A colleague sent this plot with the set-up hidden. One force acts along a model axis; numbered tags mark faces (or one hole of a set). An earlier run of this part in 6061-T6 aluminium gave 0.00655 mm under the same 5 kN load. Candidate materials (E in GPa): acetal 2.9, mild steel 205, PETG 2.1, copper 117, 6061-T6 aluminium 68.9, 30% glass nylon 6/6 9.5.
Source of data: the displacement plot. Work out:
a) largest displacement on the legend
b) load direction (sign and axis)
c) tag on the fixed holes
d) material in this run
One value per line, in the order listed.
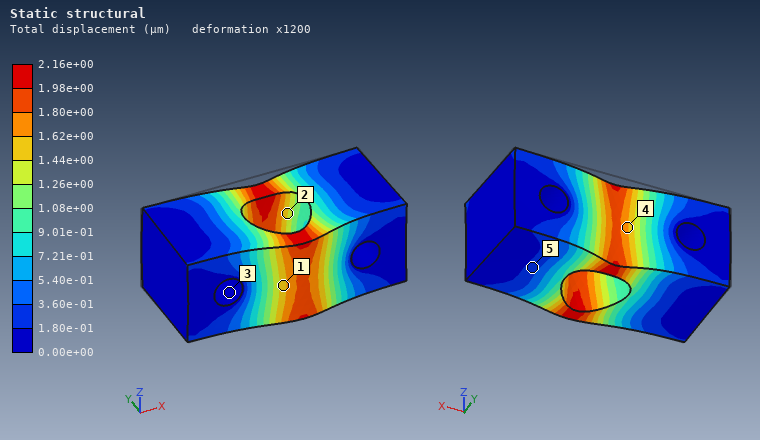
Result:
2.16e+00 µm
-Y
3
mild steel
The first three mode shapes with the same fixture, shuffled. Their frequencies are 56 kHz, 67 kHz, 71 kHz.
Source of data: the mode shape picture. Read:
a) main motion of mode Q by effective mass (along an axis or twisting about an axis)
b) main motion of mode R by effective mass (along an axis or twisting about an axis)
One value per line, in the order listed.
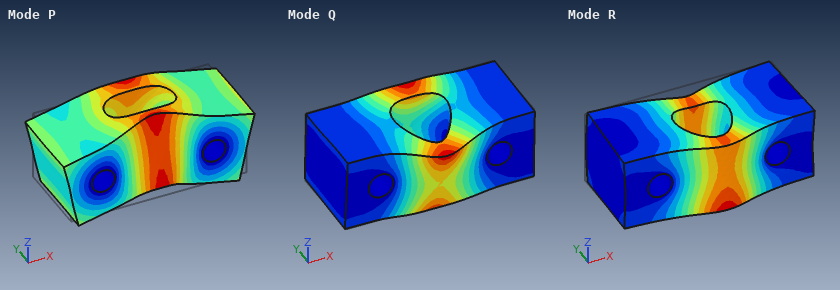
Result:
twisting about X
along Y
